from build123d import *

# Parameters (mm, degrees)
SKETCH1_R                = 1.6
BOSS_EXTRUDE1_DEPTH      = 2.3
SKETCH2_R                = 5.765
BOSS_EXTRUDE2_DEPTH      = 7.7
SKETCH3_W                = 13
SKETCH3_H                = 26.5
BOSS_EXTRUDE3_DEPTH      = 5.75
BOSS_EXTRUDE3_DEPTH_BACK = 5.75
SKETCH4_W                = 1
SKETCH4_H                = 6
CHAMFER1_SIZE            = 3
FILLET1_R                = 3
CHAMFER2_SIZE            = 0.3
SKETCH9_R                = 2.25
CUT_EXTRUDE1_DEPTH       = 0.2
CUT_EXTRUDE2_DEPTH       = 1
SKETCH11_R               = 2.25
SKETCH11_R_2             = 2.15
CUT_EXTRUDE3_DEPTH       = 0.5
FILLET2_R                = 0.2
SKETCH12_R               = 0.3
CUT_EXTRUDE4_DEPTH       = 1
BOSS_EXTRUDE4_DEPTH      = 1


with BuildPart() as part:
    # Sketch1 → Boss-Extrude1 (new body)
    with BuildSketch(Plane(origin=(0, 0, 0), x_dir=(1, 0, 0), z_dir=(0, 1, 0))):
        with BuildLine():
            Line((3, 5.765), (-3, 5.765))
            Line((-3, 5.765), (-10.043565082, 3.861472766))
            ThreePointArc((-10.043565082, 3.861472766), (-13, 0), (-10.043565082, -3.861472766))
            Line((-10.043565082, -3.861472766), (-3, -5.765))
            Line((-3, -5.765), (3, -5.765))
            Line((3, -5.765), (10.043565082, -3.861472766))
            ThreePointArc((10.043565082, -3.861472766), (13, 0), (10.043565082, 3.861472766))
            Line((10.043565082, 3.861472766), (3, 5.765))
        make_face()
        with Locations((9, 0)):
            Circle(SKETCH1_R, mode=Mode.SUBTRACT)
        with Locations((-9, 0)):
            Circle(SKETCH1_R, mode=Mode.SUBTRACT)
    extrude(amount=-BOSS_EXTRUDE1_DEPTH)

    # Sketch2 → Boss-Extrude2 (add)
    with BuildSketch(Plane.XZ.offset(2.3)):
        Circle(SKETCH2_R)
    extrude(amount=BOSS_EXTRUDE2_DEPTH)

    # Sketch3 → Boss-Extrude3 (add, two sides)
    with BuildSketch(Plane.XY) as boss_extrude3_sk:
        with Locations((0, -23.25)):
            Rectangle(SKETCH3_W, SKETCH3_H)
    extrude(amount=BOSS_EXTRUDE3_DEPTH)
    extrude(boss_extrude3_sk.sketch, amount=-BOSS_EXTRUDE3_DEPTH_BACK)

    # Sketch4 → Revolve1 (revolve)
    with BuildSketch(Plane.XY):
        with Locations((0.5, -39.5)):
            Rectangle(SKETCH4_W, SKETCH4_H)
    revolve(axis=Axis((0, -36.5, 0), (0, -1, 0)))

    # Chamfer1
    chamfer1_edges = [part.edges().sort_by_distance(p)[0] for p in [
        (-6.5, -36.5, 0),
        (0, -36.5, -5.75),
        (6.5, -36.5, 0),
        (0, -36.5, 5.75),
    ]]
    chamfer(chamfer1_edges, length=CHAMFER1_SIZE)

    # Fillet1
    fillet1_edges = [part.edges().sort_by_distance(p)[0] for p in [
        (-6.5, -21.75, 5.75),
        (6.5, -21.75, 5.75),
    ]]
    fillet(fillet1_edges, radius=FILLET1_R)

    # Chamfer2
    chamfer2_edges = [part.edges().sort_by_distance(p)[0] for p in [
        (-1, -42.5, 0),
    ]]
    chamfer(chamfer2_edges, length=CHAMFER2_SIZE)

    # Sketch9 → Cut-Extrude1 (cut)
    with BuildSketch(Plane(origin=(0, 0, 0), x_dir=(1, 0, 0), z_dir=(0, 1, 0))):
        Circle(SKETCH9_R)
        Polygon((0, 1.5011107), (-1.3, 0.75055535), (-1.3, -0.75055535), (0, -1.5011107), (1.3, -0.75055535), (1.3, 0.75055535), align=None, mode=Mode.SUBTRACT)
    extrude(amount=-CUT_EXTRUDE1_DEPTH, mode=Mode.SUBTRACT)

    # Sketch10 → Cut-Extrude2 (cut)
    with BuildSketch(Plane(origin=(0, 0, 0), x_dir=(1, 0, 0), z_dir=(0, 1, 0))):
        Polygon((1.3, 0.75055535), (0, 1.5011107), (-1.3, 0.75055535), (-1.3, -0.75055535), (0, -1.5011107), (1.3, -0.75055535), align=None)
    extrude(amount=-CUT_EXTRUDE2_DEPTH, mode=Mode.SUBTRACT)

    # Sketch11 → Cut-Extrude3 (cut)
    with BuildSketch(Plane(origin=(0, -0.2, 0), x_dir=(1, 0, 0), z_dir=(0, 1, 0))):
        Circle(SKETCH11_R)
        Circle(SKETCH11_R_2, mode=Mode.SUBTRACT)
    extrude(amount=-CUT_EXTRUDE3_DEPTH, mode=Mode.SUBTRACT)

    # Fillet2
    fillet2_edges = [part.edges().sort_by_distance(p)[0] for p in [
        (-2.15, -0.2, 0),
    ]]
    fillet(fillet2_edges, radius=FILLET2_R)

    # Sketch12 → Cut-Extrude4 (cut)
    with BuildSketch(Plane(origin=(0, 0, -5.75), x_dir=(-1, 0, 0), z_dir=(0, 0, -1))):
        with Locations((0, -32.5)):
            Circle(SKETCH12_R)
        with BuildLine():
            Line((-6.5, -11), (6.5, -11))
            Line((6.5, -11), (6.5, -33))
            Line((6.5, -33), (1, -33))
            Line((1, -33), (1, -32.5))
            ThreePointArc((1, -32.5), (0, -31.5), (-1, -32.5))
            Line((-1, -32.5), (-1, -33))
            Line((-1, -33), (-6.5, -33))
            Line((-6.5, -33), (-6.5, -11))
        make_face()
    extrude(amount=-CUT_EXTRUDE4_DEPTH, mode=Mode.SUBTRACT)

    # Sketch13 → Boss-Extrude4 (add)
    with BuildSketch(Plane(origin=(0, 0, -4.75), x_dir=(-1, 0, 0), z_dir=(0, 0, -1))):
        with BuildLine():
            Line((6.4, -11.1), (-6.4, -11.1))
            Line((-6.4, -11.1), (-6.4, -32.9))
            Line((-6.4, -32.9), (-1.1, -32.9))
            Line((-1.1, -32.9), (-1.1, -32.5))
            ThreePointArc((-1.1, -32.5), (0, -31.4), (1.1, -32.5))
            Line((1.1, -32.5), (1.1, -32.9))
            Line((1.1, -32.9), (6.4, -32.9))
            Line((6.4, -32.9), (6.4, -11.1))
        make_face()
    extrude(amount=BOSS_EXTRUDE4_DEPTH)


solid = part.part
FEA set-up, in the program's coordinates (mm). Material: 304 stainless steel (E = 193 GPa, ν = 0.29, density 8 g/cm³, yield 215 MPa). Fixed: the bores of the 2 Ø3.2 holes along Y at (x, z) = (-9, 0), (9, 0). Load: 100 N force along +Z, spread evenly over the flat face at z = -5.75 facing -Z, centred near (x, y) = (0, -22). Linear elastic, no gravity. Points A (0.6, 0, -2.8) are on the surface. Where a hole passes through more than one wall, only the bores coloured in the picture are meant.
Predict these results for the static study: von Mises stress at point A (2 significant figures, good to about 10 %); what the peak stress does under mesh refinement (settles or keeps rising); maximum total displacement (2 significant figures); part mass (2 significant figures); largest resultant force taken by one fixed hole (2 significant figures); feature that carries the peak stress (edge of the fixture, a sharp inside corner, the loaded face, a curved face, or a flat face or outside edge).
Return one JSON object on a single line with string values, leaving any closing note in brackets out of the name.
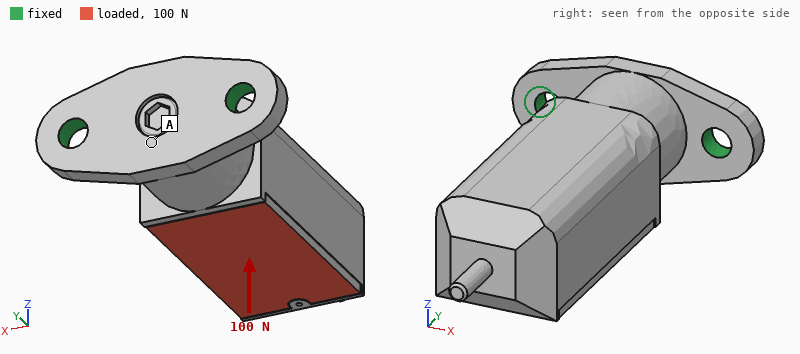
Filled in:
{"von Mises stress at point A": "14 MPa", "what the peak stress does under mesh refinement": "keeps rising", "maximum total displacement": "51 µm", "part mass": "40 g", "largest resultant force taken by one fixed hole": "50 N", "feature that carries the peak stress": "edge of the fixture"}
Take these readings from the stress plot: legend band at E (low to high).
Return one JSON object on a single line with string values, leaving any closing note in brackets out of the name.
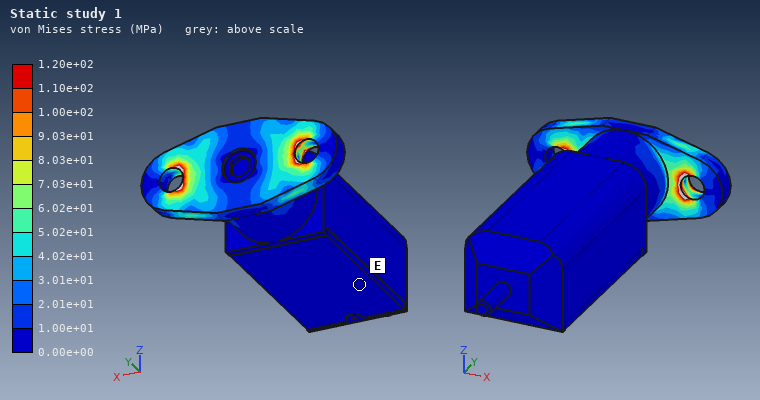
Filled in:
{"legend band at E": "0.00e+00 to 1.00e+01 MPa"}
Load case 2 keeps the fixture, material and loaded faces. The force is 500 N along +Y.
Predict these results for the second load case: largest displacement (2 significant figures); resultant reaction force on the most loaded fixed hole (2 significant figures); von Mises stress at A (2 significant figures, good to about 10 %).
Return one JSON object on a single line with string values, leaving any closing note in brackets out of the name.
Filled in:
{"largest displacement": "73 µm", "resultant reaction force on the most loaded fixed hole": "270 N", "von Mises stress at A": "27 MPa"}
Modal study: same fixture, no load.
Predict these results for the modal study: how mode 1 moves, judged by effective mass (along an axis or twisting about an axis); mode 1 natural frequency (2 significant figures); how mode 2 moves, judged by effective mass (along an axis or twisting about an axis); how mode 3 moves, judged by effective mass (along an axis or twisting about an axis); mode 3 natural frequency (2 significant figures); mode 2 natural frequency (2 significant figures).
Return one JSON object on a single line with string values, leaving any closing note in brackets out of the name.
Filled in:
{"how mode 1 moves, judged by effective mass": "along Z", "mode 1 natural frequency": "1600 Hz", "how mode 2 moves, judged by effective mass": "along X", "how mode 3 moves, judged by effective mass": "along Y", "mode 3 natural frequency": "14 kHz", "mode 2 natural frequency": "3900 Hz"}
